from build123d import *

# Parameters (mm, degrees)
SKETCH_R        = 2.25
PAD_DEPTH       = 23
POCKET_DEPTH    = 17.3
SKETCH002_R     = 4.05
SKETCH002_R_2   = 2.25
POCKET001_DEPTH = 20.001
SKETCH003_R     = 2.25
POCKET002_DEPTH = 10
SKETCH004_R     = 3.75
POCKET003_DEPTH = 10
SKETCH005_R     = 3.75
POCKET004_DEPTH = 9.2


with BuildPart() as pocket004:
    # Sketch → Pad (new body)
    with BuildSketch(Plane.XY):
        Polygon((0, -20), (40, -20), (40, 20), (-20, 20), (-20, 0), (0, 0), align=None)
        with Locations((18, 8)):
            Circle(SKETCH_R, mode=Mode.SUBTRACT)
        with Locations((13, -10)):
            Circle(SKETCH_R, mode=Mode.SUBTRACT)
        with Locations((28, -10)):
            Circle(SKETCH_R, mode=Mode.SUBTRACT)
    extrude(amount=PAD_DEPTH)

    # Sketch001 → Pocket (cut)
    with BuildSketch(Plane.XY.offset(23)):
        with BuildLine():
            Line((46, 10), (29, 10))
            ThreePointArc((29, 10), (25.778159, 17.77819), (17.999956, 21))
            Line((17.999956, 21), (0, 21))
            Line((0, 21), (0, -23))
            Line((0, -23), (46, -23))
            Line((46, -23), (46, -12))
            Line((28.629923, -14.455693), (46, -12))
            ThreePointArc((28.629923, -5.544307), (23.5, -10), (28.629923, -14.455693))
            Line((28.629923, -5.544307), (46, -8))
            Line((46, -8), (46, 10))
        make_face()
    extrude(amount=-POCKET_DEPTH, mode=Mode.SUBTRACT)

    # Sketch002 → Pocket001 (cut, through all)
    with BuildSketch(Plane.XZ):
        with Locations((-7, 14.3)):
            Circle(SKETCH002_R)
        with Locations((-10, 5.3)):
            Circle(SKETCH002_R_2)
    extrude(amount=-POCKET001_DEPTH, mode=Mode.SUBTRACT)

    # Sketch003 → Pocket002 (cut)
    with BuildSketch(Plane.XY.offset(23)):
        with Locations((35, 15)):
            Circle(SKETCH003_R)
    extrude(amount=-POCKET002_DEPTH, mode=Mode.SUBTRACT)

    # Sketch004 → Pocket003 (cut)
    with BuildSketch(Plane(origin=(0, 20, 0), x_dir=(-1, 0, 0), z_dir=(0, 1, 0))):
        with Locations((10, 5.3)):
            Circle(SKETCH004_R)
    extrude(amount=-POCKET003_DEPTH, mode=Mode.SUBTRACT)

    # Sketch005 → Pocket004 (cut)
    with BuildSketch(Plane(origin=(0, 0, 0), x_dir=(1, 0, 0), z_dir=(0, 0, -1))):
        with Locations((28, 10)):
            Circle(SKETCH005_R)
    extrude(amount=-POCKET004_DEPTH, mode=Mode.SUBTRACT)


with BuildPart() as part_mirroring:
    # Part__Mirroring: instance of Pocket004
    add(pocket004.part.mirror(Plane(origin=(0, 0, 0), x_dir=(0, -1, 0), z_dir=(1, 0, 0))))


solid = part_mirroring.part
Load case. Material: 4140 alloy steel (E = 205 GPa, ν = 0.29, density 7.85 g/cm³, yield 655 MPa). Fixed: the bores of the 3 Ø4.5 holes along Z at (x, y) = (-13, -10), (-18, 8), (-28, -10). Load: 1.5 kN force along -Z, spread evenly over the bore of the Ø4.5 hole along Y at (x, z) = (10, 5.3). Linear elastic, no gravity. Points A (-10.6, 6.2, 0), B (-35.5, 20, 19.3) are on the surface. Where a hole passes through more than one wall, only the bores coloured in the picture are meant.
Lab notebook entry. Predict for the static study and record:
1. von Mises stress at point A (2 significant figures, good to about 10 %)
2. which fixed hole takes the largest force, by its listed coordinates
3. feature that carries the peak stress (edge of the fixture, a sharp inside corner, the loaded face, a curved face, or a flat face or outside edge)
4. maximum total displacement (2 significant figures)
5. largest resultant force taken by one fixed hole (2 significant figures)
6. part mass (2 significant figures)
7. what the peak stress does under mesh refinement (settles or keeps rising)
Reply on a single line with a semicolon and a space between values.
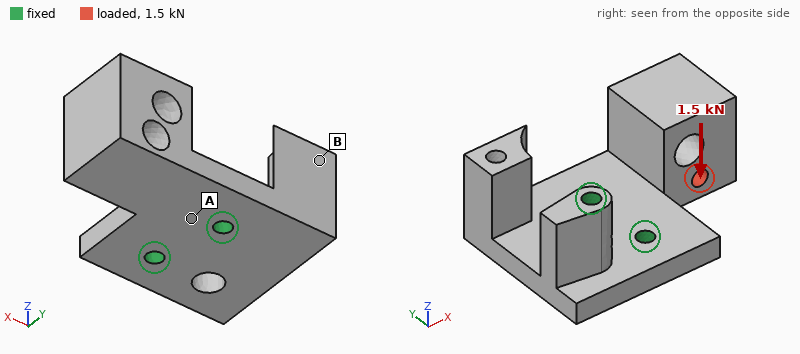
160 MPa; (-13, -10); edge of the fixture; 0.20 mm; 1.1 kN; 160 g; keeps rising
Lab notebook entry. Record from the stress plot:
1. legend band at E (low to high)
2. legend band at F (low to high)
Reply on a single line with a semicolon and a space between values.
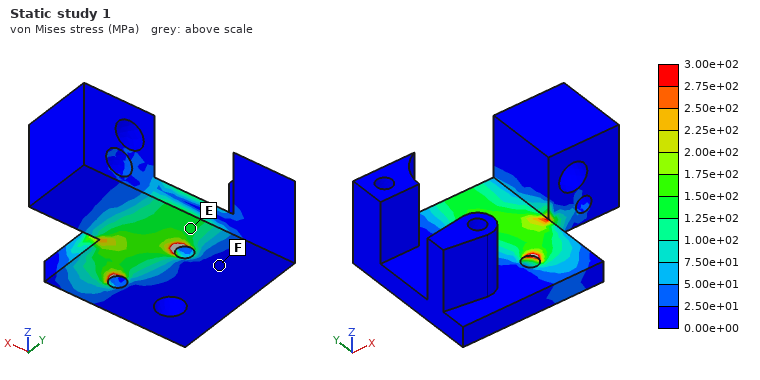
1.25e+02 to 1.50e+02 MPa; 0.00e+00 to 2.50e+01 MPa
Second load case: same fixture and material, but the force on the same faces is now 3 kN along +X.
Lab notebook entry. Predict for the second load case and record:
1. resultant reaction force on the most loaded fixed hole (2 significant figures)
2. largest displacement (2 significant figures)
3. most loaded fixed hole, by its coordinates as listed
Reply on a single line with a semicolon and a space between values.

2.4 kN; 58 µm; (-18, 8)
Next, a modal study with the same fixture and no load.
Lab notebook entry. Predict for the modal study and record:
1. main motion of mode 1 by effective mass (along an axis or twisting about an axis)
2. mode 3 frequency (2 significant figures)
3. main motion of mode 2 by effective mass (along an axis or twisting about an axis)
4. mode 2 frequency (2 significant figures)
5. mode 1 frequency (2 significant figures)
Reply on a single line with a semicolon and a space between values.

along Z; 5400 Hz; along Y; 4500 Hz; 1900 Hz
